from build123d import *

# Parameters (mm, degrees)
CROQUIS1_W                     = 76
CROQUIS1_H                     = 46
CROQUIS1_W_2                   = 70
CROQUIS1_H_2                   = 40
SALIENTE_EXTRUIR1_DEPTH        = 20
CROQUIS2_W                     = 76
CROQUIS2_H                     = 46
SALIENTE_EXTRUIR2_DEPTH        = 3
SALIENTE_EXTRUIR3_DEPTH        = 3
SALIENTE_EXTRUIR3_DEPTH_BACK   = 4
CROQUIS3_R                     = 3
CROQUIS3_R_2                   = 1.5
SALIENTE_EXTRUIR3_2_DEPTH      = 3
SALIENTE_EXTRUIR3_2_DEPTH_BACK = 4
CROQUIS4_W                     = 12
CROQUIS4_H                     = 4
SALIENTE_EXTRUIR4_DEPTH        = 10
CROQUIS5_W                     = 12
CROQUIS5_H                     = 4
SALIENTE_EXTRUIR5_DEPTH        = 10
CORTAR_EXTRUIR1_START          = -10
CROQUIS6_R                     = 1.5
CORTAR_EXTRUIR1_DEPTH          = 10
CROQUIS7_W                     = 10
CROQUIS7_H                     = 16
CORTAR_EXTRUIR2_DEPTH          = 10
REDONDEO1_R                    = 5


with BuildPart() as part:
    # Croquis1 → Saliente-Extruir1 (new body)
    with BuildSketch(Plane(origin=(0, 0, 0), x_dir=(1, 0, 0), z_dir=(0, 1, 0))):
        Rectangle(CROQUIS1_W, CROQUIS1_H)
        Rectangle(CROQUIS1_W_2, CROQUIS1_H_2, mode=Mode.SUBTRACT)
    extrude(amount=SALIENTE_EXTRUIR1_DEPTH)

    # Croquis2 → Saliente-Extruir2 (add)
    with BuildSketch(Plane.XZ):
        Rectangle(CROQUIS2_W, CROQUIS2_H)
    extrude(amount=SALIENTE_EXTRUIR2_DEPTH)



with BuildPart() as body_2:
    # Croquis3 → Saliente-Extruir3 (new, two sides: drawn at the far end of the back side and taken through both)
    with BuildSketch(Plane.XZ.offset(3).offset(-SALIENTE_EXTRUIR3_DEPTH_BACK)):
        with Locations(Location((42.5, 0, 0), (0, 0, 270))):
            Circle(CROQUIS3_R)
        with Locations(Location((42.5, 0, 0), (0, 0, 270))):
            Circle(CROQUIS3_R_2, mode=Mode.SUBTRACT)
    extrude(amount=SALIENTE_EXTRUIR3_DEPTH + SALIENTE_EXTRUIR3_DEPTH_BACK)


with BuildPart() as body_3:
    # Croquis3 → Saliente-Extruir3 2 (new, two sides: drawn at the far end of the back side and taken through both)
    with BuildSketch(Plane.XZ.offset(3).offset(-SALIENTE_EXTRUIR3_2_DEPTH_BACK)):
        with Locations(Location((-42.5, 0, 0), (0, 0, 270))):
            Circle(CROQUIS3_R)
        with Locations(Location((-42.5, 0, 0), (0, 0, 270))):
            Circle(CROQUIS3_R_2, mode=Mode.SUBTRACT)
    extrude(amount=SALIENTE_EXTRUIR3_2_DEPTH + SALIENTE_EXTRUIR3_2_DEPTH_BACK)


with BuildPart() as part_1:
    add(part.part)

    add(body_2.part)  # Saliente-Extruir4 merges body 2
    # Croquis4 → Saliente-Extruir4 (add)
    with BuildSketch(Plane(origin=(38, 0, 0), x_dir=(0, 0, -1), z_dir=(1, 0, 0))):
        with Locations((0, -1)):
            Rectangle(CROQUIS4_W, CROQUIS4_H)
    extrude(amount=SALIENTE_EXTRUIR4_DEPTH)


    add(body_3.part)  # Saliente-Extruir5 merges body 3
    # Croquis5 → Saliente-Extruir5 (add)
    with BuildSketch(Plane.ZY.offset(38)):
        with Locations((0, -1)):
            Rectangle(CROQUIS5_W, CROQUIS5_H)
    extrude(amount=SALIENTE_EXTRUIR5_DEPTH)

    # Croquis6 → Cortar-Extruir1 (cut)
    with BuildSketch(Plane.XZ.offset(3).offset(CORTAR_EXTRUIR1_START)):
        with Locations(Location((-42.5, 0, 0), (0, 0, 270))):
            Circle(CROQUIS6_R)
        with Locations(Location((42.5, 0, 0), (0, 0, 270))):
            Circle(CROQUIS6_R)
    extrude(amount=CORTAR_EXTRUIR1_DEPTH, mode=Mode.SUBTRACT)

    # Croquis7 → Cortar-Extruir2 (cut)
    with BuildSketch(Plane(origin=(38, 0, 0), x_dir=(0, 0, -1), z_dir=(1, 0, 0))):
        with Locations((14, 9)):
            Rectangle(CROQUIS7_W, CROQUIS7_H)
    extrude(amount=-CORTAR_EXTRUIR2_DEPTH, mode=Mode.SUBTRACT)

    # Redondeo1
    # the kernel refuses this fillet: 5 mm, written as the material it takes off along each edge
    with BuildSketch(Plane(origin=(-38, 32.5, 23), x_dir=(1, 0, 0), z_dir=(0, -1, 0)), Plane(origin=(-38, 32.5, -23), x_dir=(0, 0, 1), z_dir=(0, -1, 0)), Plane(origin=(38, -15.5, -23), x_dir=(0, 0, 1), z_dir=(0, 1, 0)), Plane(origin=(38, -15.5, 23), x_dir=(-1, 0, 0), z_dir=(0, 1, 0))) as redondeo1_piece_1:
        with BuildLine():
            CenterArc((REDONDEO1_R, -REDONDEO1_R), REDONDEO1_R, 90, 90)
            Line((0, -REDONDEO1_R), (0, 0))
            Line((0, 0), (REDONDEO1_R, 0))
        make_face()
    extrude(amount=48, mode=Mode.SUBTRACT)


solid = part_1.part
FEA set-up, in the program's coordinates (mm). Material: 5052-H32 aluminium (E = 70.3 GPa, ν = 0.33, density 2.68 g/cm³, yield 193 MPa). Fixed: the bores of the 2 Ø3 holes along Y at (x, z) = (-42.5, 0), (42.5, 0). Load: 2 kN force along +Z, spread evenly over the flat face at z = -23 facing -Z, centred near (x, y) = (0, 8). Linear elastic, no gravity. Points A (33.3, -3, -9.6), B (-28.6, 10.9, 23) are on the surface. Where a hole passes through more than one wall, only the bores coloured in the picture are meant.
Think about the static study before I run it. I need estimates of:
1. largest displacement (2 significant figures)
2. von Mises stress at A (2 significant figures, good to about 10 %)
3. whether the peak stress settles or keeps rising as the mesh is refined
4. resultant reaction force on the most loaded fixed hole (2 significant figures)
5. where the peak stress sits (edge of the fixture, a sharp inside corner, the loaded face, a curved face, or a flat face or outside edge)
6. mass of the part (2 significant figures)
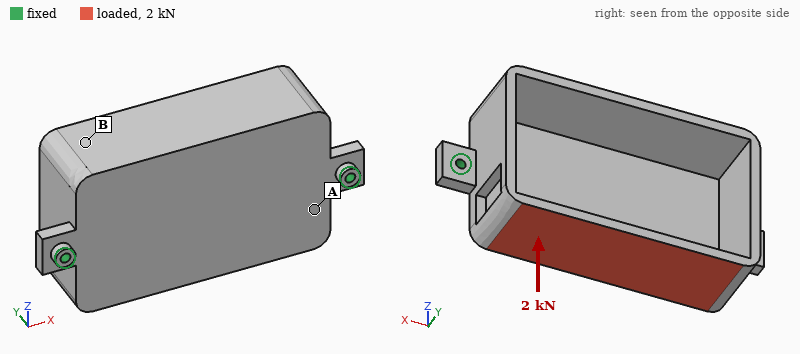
0.52 mm
52 MPa
keeps rising
1.0 kN
edge of the fixture
66 g
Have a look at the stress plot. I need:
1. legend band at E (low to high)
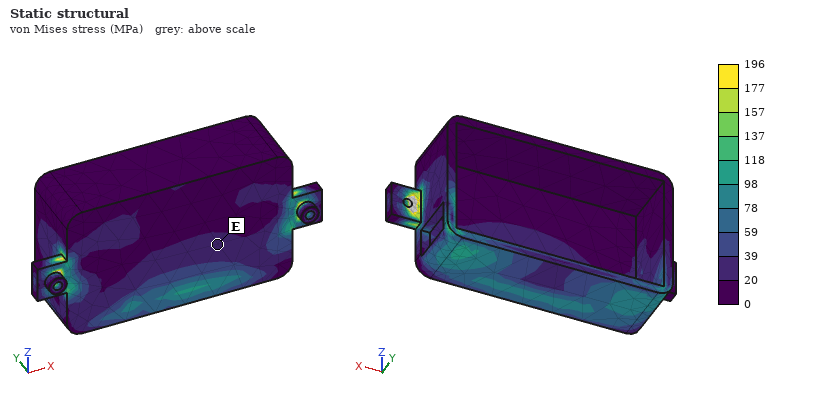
20 to 39 MPa
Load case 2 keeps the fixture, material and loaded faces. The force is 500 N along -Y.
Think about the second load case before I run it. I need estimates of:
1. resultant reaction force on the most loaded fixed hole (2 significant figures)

250 N
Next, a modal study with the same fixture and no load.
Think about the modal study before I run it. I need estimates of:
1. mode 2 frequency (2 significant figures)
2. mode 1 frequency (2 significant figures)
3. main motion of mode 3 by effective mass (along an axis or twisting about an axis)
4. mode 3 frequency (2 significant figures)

3200 Hz
1700 Hz
along Y
4100 Hz
